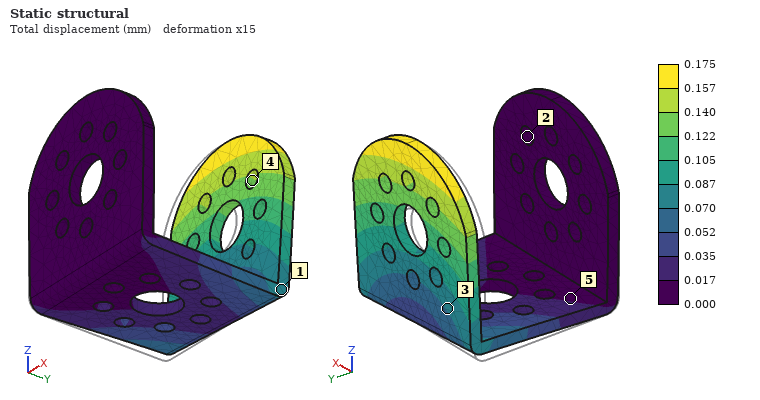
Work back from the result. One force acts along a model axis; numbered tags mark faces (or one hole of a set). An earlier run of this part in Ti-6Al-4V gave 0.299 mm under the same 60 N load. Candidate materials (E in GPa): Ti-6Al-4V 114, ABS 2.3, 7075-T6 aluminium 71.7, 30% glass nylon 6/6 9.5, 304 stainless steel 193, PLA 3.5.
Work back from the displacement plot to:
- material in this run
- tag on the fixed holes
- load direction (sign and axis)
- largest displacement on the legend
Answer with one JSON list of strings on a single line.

["304 stainless steel", "2", "+X", "0.175 mm"]
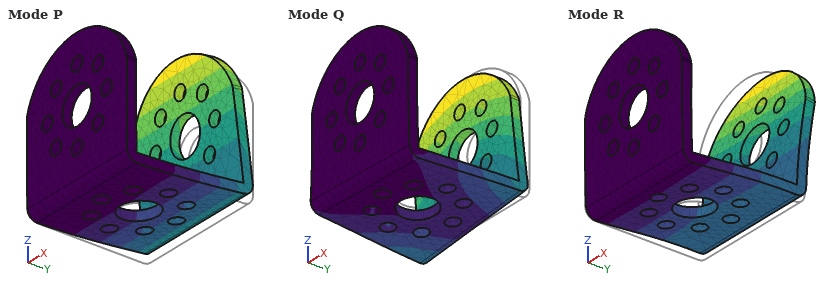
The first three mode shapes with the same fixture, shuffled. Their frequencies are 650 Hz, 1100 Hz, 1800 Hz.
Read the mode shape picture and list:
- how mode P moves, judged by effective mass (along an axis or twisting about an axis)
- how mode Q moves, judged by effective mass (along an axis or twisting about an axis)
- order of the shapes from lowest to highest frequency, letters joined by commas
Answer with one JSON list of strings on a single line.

["along Z", "along X", "P, Q, R"]
